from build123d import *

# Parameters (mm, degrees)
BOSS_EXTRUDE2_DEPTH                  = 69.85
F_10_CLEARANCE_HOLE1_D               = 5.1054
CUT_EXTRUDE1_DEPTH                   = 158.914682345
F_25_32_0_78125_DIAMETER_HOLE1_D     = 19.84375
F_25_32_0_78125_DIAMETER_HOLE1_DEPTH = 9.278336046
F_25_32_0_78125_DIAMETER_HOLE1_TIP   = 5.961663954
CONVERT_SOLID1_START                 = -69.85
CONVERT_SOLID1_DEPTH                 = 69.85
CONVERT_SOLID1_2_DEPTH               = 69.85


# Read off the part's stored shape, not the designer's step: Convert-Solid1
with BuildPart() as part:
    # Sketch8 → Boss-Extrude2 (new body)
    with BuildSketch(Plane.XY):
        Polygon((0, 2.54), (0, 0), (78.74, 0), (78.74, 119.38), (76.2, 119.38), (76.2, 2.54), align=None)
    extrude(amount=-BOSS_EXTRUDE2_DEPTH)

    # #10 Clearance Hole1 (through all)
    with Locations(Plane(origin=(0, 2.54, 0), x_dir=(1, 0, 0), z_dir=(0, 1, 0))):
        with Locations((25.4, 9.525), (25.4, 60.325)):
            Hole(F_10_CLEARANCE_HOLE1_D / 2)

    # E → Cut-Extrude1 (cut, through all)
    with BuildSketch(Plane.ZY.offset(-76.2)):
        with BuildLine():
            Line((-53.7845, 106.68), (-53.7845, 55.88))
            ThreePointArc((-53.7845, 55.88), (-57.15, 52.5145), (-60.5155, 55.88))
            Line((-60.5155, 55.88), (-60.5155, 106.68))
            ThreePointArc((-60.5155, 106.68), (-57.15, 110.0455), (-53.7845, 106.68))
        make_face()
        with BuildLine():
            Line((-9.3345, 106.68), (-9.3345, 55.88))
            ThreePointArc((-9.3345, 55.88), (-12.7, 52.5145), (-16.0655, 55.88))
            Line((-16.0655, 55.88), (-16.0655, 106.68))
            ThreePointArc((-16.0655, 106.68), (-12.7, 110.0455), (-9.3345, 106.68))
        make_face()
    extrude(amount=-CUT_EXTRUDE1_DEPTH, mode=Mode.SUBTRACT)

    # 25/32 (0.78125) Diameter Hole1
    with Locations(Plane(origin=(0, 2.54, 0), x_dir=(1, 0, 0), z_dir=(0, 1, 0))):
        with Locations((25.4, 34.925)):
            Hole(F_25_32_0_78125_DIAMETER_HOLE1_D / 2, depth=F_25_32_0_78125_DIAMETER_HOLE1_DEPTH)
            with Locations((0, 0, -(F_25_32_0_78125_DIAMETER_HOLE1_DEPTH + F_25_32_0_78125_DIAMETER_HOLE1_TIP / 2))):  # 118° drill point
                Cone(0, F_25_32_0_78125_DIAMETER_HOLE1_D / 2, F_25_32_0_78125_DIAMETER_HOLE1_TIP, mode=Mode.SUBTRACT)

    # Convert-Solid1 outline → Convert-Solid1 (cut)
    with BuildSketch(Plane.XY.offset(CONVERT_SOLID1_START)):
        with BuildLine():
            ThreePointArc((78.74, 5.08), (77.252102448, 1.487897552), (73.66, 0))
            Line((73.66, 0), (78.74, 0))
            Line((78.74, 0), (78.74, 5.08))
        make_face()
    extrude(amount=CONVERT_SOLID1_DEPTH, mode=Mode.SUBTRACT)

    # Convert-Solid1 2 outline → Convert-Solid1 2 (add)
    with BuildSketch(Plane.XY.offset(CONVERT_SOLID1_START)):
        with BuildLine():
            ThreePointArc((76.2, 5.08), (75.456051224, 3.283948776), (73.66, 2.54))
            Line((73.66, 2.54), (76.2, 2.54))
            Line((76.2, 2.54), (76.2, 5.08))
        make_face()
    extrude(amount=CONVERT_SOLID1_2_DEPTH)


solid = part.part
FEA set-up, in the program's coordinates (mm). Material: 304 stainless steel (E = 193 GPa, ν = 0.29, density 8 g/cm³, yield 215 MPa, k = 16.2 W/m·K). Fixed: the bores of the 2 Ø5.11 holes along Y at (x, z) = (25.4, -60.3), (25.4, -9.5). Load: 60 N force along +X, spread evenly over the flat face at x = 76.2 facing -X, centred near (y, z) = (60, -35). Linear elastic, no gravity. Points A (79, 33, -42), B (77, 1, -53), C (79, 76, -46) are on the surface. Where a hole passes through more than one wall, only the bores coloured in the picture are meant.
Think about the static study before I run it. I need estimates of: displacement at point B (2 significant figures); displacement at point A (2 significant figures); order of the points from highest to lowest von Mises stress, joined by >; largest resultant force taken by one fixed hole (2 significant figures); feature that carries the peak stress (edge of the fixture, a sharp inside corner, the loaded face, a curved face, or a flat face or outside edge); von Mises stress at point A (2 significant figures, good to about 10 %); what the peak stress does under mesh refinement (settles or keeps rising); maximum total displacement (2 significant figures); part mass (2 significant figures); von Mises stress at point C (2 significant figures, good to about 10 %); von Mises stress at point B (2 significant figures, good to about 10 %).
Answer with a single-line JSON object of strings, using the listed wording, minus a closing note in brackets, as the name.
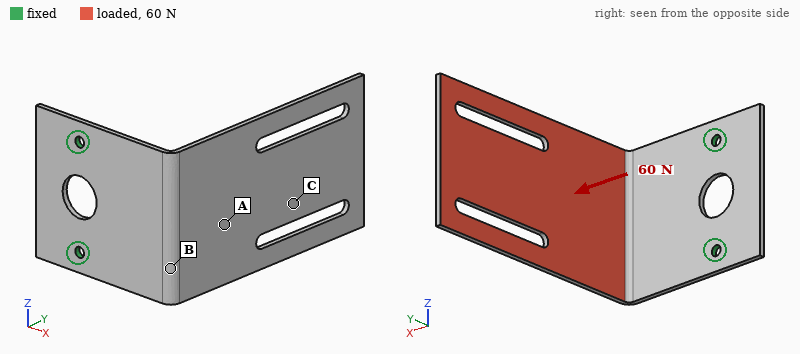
{"displacement at point B": "0.28 mm", "displacement at point A": "0.50 mm", "order of the points from highest to lowest von Mises stress, joined by >": "B > A > C", "largest resultant force taken by one fixed hole": "32 N", "feature that carries the peak stress": "edge of the fixture", "von Mises stress at point A": "22 MPa", "what the peak stress does under mesh refinement": "keeps rising", "maximum total displacement": "1.9 mm", "part mass": "250 g", "von Mises stress at point C": "8.1 MPa", "von Mises stress at point B": "35 MPa"}
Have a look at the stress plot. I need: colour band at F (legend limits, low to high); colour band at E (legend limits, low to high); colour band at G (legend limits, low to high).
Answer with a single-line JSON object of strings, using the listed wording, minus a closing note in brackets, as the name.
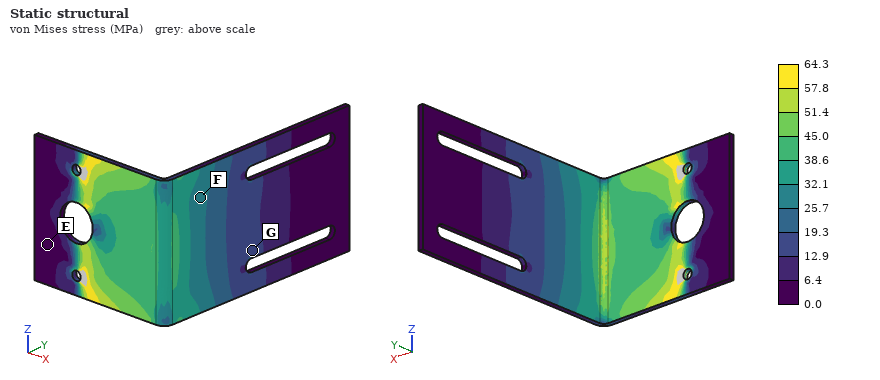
{"colour band at F": "25.7 to 32.1 MPa", "colour band at E": "0.0 to 6.4 MPa", "colour band at G": "12.9 to 19.3 MPa"}
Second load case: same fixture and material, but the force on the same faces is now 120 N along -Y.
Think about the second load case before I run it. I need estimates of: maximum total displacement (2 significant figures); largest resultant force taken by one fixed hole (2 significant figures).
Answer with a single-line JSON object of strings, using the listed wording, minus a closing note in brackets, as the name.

{"maximum total displacement": "1.1 mm", "largest resultant force taken by one fixed hole": "60 N"}
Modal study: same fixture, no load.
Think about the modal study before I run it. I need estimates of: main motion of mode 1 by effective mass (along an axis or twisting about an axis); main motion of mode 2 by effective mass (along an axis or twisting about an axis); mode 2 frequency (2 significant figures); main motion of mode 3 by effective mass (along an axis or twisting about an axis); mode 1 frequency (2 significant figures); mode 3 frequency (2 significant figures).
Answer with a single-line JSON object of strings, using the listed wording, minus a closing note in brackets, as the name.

{"main motion of mode 1 by effective mass": "along X", "main motion of mode 2 by effective mass": "along Z", "mode 2 frequency": "180 Hz", "main motion of mode 3 by effective mass": "along Y", "mode 1 frequency": "89 Hz", "mode 3 frequency": "330 Hz"}
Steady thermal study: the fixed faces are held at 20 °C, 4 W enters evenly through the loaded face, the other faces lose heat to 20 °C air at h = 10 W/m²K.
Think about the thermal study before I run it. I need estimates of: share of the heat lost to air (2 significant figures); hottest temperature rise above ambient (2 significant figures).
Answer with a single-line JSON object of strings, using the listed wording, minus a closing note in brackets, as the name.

{"share of the heat lost to air": "85 %", "hottest temperature rise above ambient": "37 K"}
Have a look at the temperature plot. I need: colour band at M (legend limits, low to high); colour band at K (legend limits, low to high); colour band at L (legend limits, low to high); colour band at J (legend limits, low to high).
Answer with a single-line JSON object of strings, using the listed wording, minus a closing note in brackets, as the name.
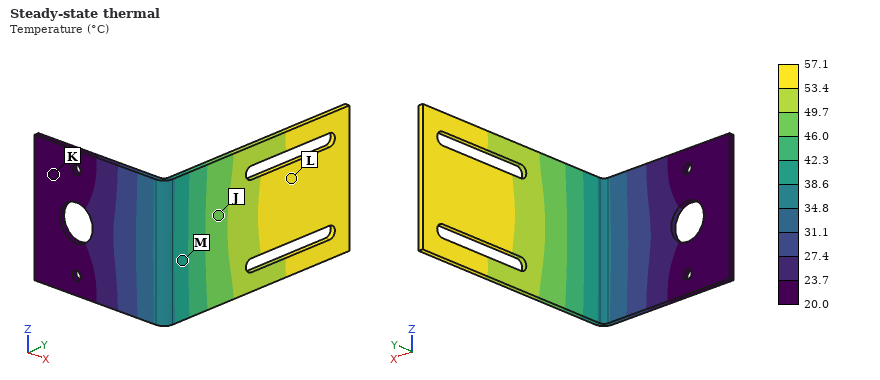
{"colour band at M": "38.6 to 42.3 °C", "colour band at K": "20.0 to 23.7 °C", "colour band at L": "53.4 to 57.1 °C", "colour band at J": "46.0 to 49.7 °C"}
